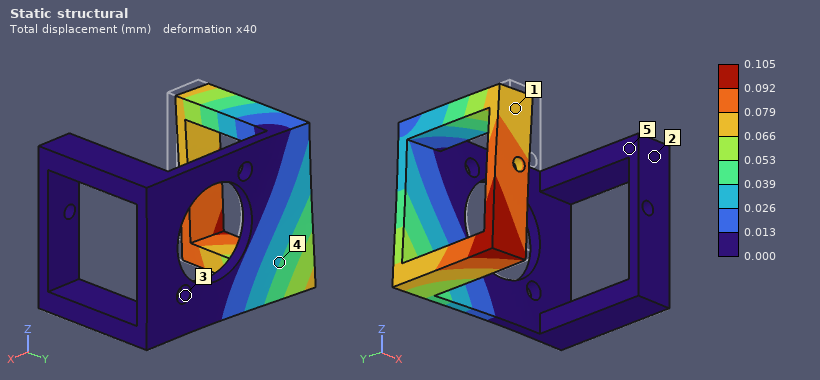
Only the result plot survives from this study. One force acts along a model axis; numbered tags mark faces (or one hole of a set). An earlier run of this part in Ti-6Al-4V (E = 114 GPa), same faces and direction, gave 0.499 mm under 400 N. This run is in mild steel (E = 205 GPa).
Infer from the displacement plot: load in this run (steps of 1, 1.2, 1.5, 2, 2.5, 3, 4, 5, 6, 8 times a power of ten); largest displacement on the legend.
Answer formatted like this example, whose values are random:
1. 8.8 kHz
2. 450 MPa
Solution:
1. 150 N
2. 0.105 mm
